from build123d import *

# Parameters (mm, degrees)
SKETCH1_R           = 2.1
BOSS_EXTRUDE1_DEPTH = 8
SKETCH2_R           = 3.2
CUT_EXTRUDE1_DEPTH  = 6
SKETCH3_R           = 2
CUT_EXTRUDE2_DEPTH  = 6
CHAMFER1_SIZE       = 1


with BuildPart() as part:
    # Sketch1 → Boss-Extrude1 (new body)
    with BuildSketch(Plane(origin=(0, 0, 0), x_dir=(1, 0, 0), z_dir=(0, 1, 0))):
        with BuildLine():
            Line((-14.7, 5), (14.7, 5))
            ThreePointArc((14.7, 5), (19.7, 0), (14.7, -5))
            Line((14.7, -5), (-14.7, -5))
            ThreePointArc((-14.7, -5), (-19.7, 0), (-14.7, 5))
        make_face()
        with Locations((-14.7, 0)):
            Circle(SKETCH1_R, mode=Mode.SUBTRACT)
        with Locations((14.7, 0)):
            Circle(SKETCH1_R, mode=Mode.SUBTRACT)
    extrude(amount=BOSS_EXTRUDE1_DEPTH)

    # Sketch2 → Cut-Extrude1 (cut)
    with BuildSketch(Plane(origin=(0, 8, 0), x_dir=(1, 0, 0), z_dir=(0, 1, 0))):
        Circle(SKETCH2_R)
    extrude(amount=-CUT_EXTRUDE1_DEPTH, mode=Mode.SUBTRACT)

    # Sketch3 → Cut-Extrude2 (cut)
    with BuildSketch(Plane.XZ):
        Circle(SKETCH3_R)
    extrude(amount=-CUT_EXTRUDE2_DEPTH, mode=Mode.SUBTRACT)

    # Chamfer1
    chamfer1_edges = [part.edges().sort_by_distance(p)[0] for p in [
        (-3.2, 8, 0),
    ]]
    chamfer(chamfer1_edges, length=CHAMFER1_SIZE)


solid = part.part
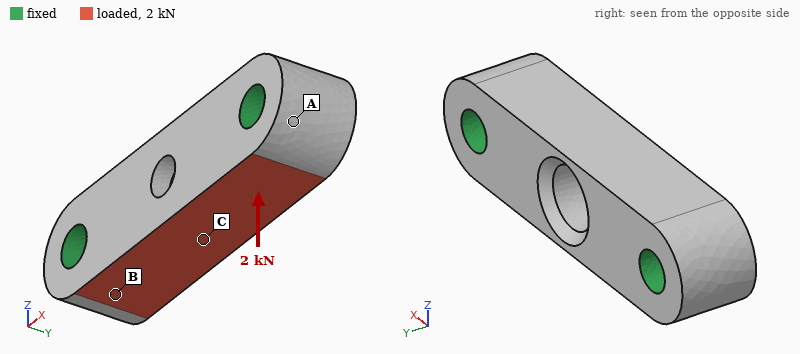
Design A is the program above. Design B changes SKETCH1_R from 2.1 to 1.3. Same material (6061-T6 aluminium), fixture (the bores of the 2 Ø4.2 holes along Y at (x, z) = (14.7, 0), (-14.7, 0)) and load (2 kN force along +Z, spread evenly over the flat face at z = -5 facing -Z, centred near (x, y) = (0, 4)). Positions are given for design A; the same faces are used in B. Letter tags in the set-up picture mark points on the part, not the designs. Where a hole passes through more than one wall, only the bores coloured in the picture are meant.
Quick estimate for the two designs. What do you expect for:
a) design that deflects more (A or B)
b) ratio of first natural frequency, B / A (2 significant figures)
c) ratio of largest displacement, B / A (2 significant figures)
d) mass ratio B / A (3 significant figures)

B
0.83
1.3
1.05
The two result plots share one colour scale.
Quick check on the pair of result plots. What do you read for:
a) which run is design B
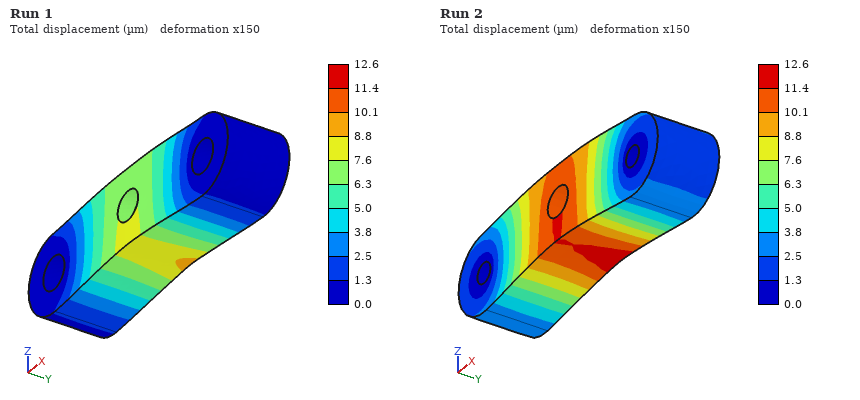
Run 2
